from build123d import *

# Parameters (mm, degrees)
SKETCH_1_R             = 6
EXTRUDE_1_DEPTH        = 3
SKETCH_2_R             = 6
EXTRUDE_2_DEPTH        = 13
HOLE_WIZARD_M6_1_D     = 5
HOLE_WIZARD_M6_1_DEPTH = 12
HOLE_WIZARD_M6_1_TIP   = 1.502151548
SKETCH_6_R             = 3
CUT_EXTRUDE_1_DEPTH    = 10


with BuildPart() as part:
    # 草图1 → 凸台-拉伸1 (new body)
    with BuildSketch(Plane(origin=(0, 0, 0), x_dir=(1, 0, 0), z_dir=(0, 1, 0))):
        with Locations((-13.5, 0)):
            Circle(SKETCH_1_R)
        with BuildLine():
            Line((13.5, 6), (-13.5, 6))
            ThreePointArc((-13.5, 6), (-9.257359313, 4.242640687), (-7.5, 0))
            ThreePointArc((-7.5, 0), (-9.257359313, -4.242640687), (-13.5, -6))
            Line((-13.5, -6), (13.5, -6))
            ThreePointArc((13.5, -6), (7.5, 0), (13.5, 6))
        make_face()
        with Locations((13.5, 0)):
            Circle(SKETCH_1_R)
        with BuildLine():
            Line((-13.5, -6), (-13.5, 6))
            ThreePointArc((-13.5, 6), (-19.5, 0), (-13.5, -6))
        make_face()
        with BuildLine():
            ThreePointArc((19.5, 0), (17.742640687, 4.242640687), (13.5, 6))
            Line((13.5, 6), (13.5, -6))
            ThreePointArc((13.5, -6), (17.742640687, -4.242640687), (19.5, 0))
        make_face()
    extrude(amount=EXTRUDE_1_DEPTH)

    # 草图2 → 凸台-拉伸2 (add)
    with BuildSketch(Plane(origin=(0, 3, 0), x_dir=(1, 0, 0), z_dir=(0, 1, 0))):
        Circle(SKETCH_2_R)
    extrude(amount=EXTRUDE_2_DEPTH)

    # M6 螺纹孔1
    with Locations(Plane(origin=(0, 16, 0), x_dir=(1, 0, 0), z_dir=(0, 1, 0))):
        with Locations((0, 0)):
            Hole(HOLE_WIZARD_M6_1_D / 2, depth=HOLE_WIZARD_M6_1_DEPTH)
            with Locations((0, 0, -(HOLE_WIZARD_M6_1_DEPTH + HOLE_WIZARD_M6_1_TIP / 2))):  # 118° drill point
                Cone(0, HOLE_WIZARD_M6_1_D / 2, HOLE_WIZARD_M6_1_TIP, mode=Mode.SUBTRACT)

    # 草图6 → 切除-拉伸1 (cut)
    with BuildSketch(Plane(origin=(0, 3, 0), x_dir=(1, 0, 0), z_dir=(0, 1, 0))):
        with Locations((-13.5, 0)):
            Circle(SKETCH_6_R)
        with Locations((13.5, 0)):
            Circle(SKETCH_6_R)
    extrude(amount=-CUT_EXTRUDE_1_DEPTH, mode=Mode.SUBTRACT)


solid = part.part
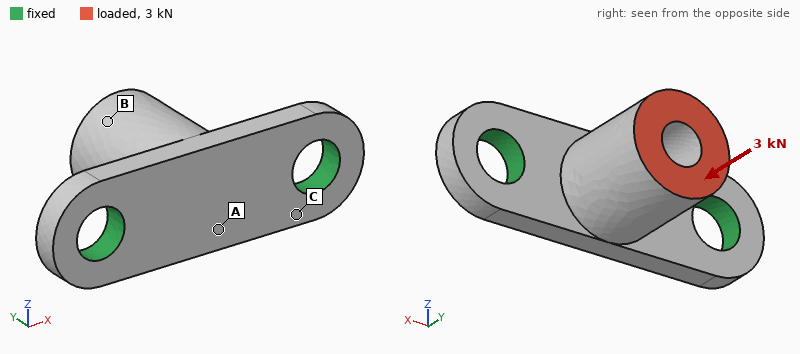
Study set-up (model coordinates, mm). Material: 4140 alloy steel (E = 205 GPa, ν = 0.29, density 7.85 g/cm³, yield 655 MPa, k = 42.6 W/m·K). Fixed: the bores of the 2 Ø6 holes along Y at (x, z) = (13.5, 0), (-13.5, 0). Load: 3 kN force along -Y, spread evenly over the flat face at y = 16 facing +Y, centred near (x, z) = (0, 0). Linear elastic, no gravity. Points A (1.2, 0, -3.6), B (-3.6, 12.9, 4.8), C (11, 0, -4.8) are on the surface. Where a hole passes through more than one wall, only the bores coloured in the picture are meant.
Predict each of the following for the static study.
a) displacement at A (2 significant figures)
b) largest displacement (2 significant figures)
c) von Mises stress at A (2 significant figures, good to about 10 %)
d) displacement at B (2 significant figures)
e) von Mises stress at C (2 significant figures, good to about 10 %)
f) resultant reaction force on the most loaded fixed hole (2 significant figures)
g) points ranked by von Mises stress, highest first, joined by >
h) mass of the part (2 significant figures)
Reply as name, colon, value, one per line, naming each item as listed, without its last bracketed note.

displacement at A: 15 µm
largest displacement: 16 µm
von Mises stress at A: 76 MPa
displacement at B: 16 µm
von Mises stress at C: 120 MPa
resultant reaction force on the most loaded fixed hole: 1.6 kN
points ranked by von Mises stress, highest first, joined by >: C > A > B
mass of the part: 19 g
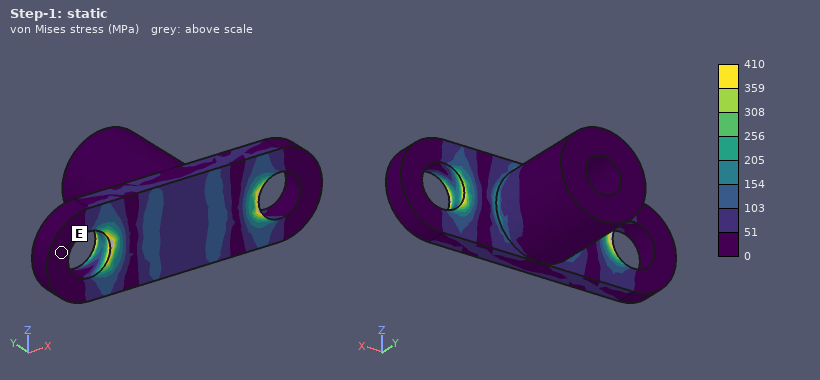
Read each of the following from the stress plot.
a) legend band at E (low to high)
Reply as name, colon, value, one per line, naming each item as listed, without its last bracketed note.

legend band at E: 0 to 51 MPa
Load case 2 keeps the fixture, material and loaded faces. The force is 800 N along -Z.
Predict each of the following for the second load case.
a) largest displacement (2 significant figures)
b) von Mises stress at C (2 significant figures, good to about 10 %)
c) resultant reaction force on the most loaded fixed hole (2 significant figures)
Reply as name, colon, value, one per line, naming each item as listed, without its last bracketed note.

largest displacement: 70 µm
von Mises stress at C: 160 MPa
resultant reaction force on the most loaded fixed hole: 400 N
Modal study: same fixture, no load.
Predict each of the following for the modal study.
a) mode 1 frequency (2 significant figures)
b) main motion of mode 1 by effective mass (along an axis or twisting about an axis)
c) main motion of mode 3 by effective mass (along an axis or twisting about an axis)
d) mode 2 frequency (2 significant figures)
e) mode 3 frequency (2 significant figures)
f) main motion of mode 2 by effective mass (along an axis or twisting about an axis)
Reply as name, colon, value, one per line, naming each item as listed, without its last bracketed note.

mode 1 frequency: 8600 Hz
main motion of mode 1 by effective mass: along Z
main motion of mode 3 by effective mass: along Y
mode 2 frequency: 18 kHz
mode 3 frequency: 19 kHz
main motion of mode 2 by effective mass: along X
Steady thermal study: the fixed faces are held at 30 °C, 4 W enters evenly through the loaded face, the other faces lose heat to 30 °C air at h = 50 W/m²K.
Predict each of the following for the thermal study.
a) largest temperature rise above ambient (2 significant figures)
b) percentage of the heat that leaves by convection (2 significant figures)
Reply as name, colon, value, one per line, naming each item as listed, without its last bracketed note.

largest temperature rise above ambient: 21 K
percentage of the heat that leaves by convection: 17 %
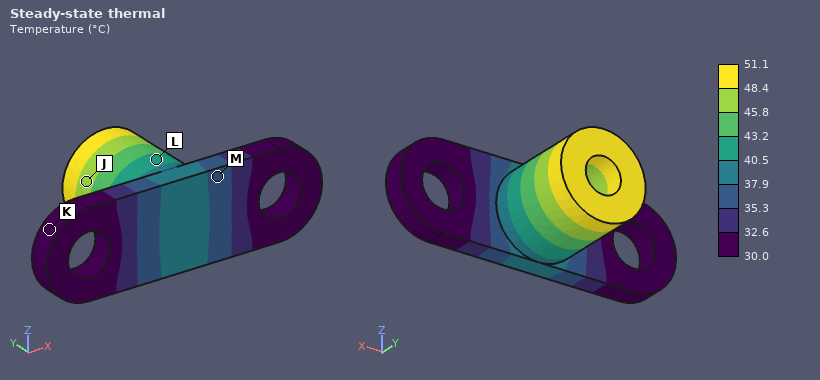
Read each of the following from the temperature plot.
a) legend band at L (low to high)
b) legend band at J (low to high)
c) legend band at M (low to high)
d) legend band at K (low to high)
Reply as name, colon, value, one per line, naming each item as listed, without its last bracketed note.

legend band at L: 40.5 to 43.2 °C
legend band at J: 45.8 to 48.4 °C
legend band at M: 35.3 to 37.9 °C
legend band at K: 30.0 to 32.6 °C
